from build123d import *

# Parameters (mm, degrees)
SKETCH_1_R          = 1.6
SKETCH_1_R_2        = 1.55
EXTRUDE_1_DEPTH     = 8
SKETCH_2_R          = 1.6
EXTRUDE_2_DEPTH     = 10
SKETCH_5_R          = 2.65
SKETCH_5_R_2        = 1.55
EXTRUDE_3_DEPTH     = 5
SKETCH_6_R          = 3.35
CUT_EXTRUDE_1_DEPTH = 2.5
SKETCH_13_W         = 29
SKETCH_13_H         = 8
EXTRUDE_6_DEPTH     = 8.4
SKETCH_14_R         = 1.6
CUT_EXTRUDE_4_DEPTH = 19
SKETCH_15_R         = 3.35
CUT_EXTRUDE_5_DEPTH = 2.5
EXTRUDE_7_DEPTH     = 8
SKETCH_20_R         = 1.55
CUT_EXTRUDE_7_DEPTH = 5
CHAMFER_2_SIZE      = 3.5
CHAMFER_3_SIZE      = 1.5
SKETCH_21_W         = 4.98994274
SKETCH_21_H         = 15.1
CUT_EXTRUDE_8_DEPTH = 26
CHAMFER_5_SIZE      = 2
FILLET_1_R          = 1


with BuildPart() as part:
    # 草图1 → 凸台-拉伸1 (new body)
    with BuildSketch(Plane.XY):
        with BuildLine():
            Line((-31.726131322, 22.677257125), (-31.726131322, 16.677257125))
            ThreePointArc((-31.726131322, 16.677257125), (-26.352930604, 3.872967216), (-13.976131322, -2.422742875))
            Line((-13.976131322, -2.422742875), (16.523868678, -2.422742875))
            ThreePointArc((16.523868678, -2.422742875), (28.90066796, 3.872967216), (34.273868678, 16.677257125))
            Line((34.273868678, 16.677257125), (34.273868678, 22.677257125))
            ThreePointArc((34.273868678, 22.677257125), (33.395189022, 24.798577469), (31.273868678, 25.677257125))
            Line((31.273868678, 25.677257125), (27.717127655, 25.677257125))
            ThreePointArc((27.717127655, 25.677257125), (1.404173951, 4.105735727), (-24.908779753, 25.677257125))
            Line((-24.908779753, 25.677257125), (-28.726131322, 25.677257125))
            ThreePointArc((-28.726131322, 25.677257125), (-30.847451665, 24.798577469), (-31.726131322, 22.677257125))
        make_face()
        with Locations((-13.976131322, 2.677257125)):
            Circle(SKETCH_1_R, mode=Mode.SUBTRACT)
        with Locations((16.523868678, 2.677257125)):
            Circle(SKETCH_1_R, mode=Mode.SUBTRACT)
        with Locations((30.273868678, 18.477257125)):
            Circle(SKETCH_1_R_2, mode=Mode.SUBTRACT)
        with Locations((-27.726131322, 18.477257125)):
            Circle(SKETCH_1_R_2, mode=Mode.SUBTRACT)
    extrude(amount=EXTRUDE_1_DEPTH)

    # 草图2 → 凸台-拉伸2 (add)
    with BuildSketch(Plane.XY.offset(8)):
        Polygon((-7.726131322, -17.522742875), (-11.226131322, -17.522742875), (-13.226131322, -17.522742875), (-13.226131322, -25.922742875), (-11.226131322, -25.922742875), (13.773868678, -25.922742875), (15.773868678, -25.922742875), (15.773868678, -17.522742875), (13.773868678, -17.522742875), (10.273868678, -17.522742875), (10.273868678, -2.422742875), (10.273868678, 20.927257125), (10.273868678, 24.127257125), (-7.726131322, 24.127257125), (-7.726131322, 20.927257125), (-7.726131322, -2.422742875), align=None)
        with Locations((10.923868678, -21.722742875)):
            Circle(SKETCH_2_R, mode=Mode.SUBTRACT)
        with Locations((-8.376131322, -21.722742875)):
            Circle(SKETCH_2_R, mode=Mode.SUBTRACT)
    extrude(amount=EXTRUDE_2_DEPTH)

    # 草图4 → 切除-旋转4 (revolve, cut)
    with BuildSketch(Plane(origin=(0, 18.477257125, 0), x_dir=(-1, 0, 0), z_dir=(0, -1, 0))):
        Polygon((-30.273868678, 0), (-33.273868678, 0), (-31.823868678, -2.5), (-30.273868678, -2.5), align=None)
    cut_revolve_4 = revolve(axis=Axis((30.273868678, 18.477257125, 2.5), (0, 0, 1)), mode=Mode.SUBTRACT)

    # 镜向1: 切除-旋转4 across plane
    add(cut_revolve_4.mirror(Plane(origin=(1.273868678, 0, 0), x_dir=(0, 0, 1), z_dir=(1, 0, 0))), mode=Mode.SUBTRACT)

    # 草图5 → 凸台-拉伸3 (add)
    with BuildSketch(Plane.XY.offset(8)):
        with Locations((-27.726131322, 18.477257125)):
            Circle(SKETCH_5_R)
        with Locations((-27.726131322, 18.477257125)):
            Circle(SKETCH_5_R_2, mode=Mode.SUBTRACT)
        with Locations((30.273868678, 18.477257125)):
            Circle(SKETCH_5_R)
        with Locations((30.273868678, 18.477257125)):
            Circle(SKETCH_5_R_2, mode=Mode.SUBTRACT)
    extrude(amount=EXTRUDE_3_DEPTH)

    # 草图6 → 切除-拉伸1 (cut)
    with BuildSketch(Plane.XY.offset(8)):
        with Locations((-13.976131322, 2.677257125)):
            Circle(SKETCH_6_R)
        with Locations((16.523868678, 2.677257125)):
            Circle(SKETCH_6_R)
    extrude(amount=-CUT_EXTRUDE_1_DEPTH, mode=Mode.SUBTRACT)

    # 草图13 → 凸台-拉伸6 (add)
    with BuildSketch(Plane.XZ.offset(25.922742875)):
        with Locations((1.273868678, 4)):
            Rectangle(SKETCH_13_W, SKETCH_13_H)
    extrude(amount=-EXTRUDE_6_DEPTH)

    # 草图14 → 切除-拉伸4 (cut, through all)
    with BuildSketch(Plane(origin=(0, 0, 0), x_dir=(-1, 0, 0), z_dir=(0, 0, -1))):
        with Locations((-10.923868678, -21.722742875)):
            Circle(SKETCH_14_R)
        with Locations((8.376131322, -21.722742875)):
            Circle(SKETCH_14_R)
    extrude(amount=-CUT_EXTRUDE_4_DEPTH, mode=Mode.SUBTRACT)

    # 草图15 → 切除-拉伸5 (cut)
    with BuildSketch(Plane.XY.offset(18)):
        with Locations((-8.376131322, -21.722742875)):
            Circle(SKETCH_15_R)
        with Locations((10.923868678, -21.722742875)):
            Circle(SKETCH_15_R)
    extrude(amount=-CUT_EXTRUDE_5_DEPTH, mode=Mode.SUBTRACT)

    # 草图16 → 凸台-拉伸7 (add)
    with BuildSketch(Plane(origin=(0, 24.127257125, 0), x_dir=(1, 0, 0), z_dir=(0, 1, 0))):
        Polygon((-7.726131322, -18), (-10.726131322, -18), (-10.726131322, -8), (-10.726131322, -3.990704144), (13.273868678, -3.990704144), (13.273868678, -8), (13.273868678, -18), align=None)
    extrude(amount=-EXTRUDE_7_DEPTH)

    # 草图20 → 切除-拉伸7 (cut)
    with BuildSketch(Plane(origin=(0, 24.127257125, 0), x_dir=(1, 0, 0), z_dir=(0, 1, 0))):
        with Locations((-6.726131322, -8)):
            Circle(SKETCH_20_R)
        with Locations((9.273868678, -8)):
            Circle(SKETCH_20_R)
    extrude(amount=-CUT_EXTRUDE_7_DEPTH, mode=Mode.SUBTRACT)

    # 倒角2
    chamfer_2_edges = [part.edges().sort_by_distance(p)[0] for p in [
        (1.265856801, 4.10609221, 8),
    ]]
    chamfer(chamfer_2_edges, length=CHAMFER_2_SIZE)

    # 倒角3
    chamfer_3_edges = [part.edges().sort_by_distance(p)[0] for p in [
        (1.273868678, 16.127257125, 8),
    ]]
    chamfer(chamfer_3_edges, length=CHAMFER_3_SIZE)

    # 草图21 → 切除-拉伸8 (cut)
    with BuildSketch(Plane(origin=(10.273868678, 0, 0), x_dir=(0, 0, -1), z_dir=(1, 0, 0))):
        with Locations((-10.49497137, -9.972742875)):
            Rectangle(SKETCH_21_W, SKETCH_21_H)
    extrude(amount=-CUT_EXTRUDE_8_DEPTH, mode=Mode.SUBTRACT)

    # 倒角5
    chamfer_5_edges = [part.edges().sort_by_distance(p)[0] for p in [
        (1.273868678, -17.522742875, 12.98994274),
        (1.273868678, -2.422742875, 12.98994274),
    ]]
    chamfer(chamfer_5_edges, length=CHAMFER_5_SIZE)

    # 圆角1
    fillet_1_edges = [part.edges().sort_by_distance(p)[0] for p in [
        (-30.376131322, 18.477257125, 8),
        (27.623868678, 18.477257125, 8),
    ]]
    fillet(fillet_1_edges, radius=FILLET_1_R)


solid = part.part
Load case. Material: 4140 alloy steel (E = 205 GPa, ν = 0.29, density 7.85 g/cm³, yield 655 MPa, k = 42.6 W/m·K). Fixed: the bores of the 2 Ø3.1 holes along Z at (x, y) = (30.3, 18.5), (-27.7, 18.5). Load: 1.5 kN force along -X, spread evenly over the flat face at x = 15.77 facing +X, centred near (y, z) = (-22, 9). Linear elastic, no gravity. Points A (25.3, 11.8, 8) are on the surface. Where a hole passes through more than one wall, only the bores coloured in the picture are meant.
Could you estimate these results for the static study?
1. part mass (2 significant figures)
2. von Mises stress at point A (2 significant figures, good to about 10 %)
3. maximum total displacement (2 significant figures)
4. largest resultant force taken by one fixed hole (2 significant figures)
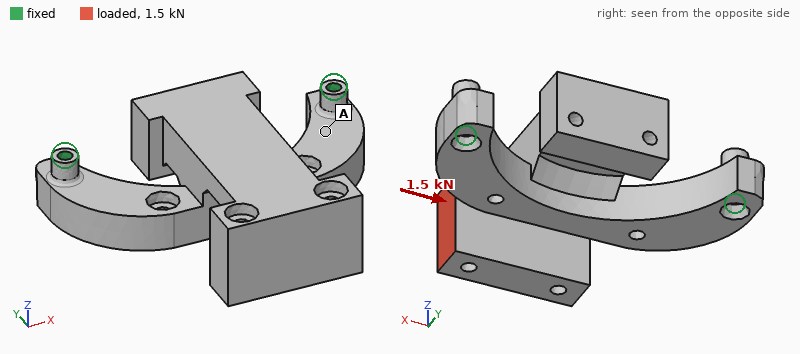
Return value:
140 g
15 MPa
0.11 mm
1.3 kN
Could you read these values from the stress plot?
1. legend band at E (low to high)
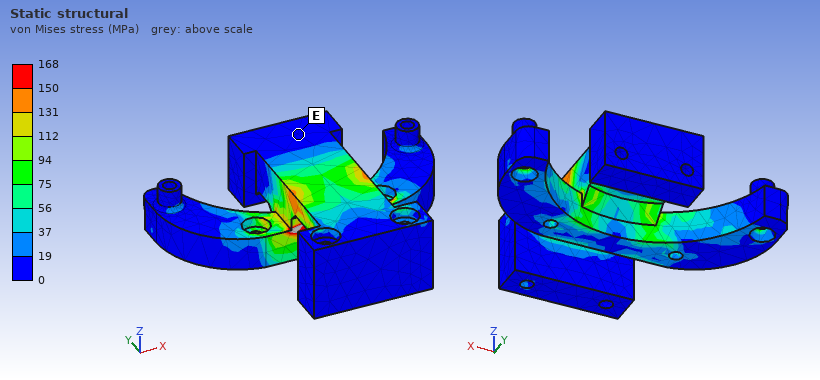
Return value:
0 to 19 MPa
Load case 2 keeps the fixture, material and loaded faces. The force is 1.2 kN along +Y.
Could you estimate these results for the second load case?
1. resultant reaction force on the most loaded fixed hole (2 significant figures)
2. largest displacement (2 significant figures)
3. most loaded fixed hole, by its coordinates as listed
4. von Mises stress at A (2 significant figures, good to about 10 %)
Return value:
1.2 kN
89 µm
(30.3, 18.5)
45 MPa
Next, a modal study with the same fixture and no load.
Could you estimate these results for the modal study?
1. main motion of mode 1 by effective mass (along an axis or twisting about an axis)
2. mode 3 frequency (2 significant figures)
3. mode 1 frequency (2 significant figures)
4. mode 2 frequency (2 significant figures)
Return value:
along Z
3500 Hz
1400 Hz
3400 Hz
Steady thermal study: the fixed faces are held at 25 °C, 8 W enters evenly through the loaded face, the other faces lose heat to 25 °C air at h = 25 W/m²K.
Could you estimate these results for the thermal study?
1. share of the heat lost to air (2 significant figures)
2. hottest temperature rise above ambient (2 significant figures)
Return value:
58 %
66 K
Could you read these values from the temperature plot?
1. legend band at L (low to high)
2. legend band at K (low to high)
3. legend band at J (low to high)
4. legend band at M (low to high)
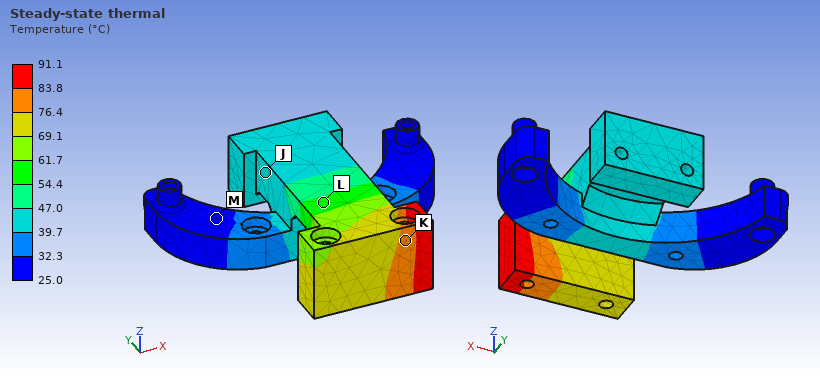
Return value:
54.4 to 61.7 °C
76.4 to 83.8 °C
39.7 to 47.0 °C
25.0 to 32.3 °C
